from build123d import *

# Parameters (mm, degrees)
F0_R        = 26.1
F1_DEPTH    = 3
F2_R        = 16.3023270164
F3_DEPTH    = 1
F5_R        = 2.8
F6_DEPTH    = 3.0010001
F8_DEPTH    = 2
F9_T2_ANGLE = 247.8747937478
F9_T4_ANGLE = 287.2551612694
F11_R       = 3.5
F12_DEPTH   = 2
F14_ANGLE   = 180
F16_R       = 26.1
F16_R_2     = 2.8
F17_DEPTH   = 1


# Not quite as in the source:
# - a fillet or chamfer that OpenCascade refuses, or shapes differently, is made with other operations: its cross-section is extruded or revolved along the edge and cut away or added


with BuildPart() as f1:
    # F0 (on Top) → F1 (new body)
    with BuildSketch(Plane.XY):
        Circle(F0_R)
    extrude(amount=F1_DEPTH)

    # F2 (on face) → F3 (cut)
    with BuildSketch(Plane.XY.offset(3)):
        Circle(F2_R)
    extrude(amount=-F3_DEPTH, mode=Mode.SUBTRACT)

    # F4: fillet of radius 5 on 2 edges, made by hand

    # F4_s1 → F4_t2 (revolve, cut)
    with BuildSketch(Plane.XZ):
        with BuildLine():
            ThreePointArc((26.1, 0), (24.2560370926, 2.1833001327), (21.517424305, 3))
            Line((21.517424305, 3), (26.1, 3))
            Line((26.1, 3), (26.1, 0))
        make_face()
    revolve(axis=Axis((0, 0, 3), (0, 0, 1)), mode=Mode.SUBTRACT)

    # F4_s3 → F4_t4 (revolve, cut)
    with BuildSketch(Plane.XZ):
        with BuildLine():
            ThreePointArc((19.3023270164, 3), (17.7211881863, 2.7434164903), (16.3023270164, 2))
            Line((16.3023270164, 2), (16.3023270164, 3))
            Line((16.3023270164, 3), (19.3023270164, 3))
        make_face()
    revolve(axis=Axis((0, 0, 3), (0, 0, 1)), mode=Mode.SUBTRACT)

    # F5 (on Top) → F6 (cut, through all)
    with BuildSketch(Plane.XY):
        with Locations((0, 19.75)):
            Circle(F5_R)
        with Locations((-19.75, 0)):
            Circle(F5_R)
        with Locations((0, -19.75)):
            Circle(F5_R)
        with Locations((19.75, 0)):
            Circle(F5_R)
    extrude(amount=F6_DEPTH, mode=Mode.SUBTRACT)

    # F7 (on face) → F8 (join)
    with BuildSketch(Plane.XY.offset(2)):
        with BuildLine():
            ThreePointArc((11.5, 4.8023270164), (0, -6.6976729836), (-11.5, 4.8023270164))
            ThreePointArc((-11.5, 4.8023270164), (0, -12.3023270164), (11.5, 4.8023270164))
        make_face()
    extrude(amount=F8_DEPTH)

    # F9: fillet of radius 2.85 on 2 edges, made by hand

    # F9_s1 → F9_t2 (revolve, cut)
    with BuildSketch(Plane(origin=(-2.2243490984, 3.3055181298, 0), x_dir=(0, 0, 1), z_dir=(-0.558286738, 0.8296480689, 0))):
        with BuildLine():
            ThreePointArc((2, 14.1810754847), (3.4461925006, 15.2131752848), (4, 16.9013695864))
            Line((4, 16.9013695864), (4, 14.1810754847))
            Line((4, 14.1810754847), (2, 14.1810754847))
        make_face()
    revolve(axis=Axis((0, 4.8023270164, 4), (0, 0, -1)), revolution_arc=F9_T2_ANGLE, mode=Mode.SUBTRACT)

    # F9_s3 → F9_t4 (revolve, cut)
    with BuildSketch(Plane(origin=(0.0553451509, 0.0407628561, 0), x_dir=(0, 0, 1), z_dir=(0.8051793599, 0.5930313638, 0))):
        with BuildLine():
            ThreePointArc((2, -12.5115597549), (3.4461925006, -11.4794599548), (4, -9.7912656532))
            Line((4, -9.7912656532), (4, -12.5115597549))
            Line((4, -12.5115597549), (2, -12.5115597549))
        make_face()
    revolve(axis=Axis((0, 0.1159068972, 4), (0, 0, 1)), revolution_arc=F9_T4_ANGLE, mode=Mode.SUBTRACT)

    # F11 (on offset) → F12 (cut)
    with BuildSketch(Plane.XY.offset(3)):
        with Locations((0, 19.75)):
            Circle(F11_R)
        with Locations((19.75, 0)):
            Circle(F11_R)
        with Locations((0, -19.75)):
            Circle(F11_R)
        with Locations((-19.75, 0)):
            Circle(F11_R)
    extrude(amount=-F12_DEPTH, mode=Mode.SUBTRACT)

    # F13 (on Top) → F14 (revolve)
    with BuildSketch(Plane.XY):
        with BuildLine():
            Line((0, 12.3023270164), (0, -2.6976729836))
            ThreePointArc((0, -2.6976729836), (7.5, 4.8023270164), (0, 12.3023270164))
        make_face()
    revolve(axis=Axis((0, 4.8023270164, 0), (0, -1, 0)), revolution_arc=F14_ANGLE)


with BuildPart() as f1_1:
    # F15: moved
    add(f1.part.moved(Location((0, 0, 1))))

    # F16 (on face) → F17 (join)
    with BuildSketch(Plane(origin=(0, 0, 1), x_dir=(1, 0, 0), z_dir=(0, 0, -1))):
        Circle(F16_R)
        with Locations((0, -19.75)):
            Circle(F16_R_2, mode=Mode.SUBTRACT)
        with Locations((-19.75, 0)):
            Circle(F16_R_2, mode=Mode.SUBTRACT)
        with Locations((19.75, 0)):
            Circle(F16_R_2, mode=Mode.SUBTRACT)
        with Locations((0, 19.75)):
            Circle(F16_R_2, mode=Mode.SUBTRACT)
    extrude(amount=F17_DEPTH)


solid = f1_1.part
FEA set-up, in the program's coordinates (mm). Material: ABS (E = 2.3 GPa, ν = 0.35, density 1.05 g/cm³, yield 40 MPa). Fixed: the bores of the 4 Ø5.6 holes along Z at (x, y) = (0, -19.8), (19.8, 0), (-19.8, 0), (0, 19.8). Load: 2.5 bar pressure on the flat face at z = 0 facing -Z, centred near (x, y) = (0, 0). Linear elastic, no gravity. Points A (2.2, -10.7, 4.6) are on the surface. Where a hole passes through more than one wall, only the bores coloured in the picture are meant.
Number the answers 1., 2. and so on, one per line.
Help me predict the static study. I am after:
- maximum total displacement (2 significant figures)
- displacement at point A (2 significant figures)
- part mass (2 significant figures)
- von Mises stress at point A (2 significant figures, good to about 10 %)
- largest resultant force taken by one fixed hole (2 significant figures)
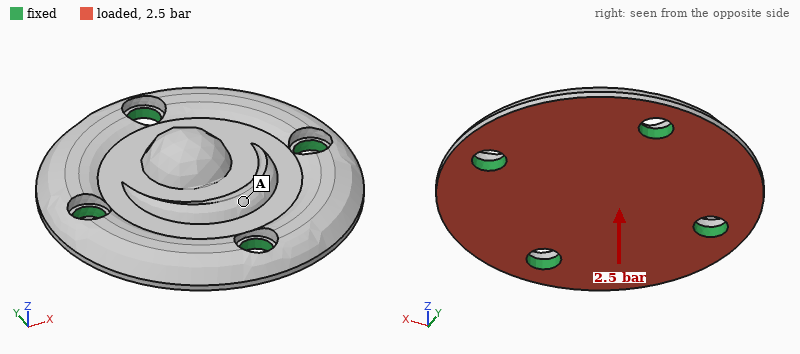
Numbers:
1. 0.13 mm
2. 0.056 mm
3. 7.6 g
4. 2.4 MPa
5. 140 N
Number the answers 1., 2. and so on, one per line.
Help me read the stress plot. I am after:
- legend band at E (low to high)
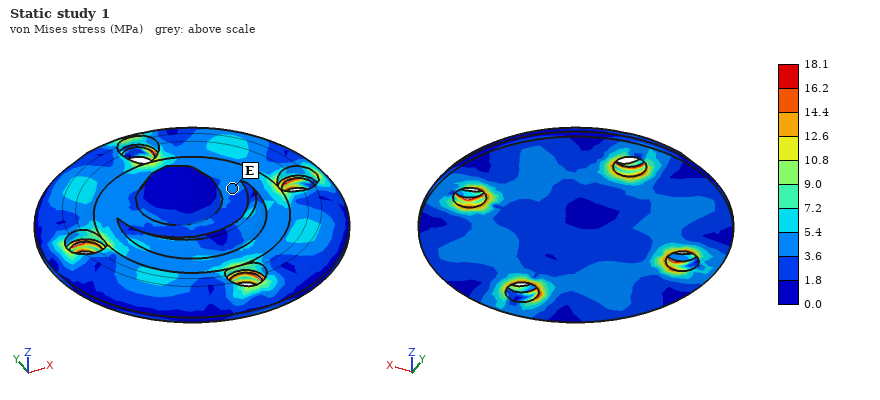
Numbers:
1. 3.6 to 5.4 MPa
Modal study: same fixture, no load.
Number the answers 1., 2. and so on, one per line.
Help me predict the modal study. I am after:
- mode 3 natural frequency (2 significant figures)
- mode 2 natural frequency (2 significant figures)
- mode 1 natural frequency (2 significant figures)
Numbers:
1. 4600 Hz
2. 4600 Hz
3. 4500 Hz
